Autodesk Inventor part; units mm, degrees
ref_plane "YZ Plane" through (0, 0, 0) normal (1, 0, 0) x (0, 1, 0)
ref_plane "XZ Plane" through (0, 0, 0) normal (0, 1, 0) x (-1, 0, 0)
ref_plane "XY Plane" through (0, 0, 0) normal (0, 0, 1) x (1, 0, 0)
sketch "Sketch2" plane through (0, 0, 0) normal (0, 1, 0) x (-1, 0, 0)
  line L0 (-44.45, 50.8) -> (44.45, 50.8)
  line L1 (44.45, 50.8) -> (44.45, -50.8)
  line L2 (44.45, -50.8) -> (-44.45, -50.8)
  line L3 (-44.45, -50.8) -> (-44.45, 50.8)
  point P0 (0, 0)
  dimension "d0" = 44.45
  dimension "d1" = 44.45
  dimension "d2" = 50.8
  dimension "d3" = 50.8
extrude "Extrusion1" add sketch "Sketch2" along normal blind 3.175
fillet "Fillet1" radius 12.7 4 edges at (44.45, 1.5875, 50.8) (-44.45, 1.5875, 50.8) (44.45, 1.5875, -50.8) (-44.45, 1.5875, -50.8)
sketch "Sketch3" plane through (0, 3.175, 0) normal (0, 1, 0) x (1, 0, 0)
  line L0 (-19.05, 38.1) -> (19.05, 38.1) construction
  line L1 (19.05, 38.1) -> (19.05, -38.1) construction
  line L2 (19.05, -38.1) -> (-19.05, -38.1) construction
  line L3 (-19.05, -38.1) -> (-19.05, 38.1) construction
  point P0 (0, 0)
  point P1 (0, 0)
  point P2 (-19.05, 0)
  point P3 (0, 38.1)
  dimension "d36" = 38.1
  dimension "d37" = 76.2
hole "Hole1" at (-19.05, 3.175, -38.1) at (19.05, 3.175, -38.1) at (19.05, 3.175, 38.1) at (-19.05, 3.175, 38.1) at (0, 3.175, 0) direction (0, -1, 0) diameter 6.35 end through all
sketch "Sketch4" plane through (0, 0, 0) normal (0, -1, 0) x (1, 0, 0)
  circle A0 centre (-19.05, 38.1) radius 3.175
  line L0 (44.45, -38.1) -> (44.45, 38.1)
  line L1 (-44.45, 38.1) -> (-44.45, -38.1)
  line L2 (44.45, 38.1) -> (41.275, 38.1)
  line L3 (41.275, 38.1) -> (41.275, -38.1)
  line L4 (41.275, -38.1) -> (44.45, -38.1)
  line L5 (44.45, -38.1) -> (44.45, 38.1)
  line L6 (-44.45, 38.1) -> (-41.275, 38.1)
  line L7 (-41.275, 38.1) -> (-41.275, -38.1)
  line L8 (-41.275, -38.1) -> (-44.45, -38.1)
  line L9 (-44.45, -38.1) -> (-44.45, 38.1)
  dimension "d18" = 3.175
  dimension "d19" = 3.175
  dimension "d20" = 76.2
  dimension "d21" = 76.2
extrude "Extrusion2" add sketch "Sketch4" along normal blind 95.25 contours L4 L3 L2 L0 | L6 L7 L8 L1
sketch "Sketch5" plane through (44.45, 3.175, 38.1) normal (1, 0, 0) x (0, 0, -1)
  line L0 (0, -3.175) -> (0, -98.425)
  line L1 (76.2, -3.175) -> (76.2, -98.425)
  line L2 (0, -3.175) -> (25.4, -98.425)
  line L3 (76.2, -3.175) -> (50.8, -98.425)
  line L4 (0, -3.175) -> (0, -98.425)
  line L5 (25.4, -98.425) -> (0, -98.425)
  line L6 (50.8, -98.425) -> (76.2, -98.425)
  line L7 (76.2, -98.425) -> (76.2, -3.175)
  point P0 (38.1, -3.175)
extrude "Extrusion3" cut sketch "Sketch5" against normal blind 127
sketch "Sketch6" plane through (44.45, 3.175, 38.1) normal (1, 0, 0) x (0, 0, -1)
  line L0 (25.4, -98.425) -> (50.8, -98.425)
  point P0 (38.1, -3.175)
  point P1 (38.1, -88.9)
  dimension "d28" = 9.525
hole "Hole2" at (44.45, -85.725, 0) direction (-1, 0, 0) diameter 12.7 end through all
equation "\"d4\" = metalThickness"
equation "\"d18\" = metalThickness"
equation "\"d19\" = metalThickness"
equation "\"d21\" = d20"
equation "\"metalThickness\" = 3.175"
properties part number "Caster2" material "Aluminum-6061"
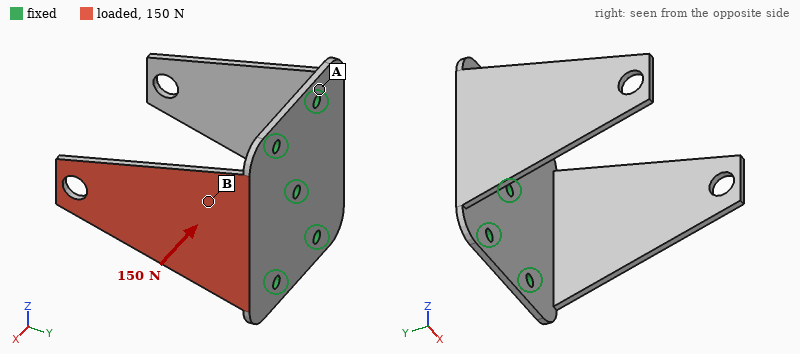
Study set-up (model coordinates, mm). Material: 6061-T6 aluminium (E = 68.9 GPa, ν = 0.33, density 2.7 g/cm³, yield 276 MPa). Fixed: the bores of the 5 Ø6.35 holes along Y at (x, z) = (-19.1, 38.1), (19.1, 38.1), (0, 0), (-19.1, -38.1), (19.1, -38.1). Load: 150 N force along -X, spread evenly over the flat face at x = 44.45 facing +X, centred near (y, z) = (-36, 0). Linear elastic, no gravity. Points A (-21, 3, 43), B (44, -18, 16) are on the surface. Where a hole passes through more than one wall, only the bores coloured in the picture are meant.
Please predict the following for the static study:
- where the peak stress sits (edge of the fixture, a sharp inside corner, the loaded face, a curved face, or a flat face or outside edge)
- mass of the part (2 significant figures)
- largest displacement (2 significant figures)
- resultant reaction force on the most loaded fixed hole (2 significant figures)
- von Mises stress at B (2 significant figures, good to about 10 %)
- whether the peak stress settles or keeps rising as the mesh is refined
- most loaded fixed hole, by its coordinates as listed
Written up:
edge of the fixture
160 g
1.6 mm
120 N
27 MPa
keeps rising
(0, 0)
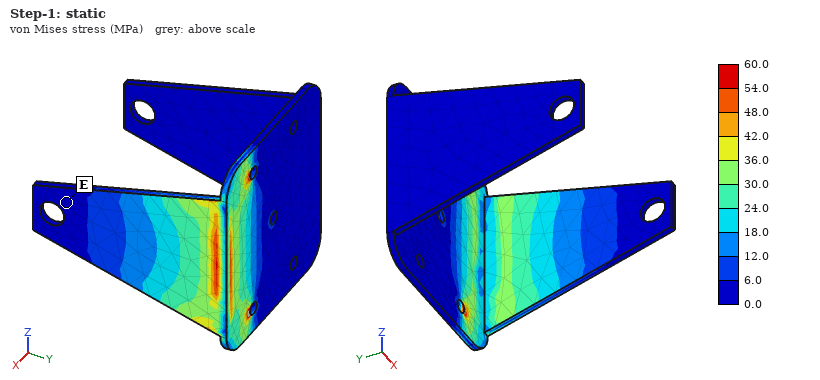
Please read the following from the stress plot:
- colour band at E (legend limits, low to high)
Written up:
0.0 to 6.0 MPa
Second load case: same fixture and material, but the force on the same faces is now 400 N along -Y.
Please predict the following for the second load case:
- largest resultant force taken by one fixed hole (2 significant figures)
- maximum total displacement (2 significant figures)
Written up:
240 N
0.81 mm
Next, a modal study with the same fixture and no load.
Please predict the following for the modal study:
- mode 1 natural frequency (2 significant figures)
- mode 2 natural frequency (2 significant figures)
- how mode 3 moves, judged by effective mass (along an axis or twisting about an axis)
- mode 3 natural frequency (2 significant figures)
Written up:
310 Hz
310 Hz
along Z
1100 Hz
